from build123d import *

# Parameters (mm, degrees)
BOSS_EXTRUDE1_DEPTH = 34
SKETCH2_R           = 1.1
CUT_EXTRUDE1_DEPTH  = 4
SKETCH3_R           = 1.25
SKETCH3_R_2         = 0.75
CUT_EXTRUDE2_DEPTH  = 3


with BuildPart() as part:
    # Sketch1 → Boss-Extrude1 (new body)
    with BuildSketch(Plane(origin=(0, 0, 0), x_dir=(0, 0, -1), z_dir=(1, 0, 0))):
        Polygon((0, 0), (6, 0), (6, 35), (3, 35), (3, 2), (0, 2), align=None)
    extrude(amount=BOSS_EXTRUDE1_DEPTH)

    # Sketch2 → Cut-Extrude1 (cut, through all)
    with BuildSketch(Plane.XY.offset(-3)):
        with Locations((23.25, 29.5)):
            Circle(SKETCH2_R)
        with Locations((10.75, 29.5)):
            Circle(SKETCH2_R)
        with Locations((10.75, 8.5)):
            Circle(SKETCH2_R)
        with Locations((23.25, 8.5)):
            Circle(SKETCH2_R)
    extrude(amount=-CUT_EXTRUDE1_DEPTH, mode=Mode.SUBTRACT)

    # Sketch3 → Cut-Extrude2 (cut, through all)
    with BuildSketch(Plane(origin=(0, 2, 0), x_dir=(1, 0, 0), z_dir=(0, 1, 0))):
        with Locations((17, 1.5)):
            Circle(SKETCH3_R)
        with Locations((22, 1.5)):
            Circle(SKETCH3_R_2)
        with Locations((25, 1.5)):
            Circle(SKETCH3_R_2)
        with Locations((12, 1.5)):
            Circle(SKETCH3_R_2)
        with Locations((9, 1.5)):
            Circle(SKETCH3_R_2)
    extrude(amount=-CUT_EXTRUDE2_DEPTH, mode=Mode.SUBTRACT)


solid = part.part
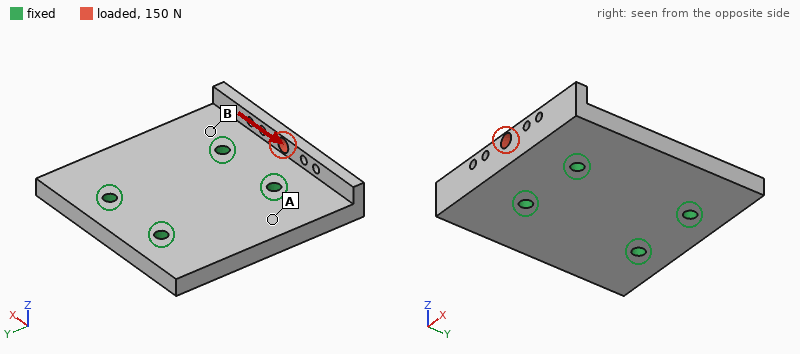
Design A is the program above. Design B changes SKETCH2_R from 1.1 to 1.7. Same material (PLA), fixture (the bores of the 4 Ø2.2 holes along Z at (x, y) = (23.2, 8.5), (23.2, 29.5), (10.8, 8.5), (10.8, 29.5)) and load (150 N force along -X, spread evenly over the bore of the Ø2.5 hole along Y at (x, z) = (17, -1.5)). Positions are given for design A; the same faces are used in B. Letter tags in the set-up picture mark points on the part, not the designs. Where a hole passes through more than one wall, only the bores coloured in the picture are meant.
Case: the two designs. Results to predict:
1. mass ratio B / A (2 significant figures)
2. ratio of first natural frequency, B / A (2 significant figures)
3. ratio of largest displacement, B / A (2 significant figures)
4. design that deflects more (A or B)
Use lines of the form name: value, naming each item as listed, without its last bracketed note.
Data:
mass ratio B / A: 0.98
ratio of first natural frequency, B / A: 1.1
ratio of largest displacement, B / A: 0.80
design that deflects more: A
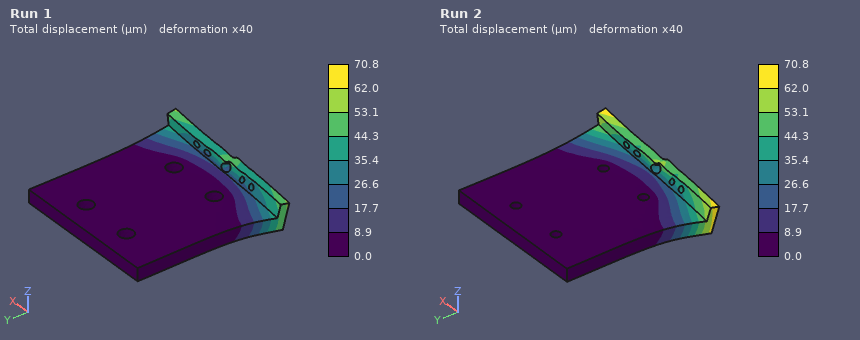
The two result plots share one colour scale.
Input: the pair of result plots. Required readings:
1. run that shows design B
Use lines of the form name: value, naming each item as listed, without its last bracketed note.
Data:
run that shows design B: Run 1
